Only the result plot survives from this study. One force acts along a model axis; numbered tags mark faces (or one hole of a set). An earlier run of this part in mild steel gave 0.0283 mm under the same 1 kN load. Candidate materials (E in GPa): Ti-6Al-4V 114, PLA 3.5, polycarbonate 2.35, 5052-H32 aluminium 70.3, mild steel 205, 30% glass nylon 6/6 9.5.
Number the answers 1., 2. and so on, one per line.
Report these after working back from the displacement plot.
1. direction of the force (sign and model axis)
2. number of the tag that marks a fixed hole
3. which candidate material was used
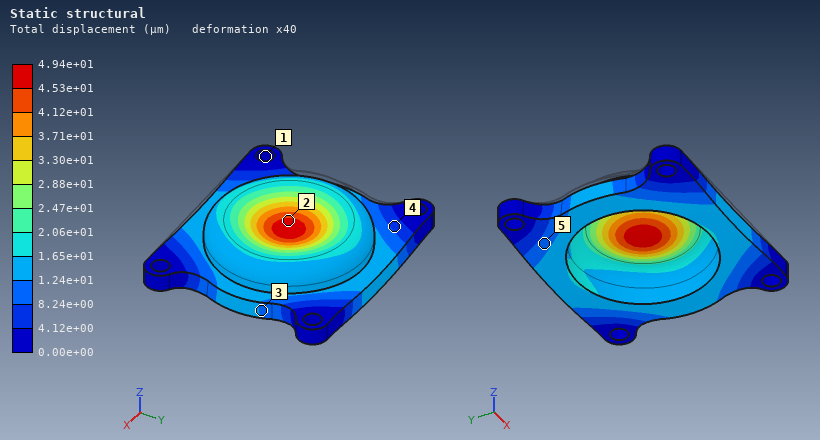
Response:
1. -Z
2. 1
3. Ti-6Al-4V
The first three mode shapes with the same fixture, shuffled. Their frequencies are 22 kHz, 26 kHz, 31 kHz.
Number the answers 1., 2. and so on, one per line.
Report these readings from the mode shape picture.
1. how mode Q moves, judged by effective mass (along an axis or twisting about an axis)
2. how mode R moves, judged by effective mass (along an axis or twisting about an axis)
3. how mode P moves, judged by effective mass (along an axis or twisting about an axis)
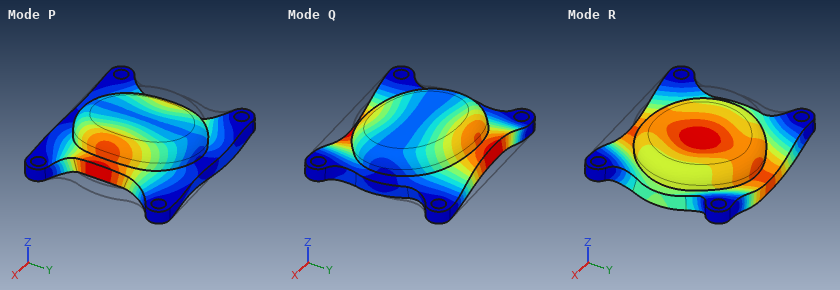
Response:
1. twisting about X
2. along Z
3. twisting about Y
